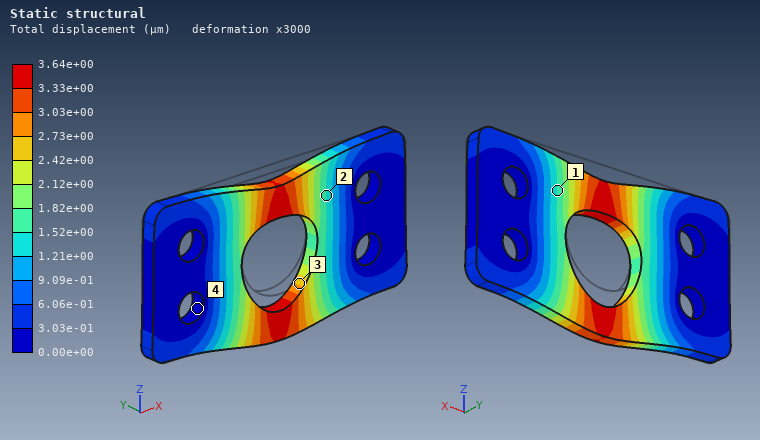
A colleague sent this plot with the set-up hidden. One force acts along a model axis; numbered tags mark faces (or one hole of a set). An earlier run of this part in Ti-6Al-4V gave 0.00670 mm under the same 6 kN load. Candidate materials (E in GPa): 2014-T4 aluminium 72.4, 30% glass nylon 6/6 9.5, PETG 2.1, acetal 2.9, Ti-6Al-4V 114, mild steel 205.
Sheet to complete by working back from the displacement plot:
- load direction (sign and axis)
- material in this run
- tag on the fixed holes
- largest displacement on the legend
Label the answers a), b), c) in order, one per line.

a) -Z
b) mild steel
c) 4
d) 3.64e+00 µm
